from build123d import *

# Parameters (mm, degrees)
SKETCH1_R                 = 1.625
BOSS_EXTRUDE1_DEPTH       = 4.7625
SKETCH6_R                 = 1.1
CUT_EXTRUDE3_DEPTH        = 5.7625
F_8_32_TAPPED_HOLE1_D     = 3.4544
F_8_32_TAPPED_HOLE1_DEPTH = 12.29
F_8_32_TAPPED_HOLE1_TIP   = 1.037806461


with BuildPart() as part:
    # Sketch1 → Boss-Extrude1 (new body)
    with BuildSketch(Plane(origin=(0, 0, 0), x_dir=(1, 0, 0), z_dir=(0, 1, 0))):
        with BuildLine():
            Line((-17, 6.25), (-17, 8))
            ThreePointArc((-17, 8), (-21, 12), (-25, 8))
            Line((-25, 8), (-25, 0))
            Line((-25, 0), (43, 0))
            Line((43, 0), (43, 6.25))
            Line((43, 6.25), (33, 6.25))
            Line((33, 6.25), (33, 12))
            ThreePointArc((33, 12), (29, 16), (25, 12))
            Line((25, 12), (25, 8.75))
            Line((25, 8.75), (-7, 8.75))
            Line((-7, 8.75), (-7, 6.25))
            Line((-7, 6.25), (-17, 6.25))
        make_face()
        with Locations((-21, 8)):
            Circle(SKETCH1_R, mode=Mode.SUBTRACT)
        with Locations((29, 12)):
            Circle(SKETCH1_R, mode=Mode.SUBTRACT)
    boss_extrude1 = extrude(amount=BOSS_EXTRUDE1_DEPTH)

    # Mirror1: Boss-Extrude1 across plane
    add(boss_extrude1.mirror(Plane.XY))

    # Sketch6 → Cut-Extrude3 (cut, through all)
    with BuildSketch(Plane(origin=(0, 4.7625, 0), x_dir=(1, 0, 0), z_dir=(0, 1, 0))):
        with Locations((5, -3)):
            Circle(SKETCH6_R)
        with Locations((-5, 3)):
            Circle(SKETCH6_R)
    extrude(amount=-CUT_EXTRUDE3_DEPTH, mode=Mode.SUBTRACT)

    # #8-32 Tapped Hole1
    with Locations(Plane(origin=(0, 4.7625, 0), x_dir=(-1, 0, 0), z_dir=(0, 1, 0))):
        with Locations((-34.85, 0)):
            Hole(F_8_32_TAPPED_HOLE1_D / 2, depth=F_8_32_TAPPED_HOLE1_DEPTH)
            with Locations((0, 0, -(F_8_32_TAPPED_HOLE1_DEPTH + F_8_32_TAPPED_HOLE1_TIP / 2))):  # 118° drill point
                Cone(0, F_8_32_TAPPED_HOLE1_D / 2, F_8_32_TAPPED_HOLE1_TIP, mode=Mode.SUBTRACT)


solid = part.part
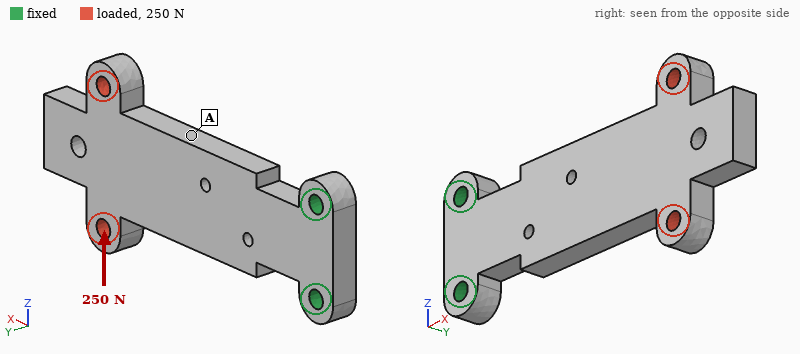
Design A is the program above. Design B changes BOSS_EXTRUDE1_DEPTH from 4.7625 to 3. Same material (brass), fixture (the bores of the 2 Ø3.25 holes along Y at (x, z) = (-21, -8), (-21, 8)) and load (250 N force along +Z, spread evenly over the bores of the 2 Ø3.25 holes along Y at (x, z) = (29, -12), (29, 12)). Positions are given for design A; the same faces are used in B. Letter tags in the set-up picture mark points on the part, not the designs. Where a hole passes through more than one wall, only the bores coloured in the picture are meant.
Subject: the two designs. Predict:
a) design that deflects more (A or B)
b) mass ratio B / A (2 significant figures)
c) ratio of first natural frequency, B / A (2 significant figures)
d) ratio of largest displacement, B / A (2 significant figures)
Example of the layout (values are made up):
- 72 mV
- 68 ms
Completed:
- B
- 0.63
- 0.64
- 1.6
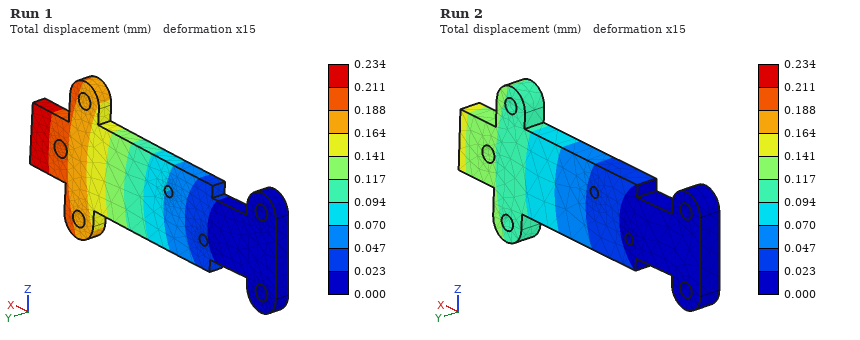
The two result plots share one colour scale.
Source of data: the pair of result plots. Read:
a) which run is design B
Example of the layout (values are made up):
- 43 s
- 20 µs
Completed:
- Run 1
